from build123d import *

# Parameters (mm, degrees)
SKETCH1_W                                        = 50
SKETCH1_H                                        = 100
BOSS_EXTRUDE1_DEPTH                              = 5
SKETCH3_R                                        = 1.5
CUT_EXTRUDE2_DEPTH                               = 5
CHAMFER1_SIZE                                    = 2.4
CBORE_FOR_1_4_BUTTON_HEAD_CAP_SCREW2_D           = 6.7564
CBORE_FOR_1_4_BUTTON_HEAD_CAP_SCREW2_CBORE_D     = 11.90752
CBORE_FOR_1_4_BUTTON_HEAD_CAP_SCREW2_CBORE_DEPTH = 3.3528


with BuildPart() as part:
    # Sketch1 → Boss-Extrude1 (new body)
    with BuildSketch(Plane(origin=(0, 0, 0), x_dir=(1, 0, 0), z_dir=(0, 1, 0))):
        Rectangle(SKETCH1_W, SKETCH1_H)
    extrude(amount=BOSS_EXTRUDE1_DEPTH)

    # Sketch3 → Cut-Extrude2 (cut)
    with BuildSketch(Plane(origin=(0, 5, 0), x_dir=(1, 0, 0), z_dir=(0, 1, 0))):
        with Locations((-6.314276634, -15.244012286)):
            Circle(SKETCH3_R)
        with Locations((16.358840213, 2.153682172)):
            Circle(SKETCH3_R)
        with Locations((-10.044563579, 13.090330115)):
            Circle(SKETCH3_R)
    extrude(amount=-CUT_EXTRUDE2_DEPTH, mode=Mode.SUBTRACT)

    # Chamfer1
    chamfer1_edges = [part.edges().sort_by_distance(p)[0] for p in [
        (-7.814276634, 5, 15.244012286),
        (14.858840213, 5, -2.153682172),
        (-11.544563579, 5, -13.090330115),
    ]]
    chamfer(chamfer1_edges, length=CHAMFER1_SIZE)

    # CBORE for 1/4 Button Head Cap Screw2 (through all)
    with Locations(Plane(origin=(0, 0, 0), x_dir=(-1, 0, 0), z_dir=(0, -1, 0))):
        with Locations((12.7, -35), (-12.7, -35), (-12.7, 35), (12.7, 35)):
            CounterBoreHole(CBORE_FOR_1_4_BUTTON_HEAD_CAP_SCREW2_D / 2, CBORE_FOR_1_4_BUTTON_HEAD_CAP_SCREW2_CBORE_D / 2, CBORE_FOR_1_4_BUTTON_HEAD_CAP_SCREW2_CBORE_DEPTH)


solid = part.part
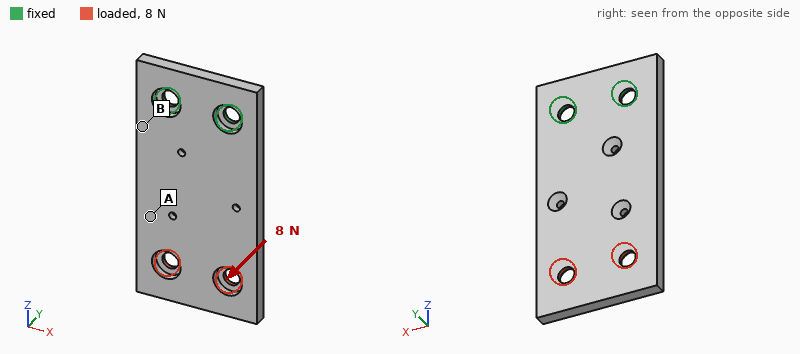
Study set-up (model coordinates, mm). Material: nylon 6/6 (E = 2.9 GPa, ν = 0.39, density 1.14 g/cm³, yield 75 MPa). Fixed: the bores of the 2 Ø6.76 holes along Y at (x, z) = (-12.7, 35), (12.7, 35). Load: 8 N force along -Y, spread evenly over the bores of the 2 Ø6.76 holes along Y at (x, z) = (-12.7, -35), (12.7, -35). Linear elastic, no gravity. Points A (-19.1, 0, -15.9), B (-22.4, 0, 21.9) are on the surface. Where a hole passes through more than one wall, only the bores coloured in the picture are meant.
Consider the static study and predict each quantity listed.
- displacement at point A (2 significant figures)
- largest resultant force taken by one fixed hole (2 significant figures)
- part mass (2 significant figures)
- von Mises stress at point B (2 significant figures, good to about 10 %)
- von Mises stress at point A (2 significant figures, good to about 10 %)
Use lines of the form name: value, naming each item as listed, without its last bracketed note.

displacement at point A: 0.60 mm
largest resultant force taken by one fixed hole: 11 N
part mass: 26 g
von Mises stress at point B: 2.5 MPa
von Mises stress at point A: 0.82 MPa
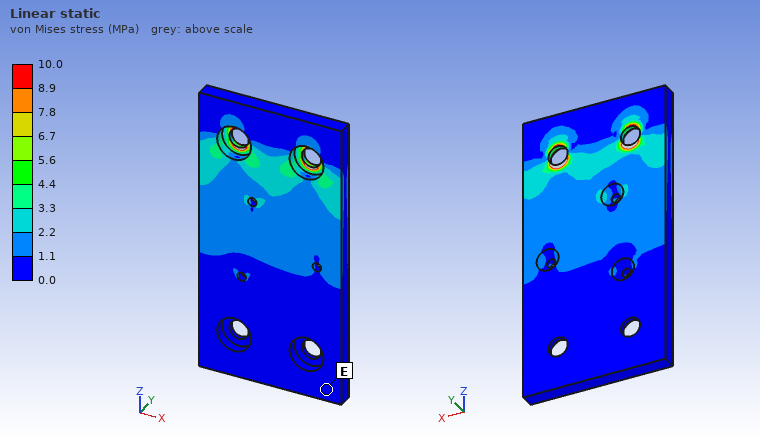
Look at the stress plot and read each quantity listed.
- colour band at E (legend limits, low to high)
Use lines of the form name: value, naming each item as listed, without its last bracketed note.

colour band at E: 0.0 to 1.1 MPa
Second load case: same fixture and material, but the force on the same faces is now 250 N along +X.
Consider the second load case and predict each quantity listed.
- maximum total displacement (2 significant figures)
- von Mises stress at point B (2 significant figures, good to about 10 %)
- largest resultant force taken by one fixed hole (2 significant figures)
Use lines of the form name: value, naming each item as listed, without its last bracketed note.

maximum total displacement: 0.89 mm
von Mises stress at point B: 4.4 MPa
largest resultant force taken by one fixed hole: 610 N
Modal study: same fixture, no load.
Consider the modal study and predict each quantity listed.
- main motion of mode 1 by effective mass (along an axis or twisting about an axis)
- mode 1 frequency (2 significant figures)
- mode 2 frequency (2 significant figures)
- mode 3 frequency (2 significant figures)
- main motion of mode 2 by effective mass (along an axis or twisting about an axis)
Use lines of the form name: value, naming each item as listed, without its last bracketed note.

main motion of mode 1 by effective mass: along Y
mode 1 frequency: 150 Hz
mode 2 frequency: 590 Hz
mode 3 frequency: 930 Hz
main motion of mode 2 by effective mass: twisting about Z
